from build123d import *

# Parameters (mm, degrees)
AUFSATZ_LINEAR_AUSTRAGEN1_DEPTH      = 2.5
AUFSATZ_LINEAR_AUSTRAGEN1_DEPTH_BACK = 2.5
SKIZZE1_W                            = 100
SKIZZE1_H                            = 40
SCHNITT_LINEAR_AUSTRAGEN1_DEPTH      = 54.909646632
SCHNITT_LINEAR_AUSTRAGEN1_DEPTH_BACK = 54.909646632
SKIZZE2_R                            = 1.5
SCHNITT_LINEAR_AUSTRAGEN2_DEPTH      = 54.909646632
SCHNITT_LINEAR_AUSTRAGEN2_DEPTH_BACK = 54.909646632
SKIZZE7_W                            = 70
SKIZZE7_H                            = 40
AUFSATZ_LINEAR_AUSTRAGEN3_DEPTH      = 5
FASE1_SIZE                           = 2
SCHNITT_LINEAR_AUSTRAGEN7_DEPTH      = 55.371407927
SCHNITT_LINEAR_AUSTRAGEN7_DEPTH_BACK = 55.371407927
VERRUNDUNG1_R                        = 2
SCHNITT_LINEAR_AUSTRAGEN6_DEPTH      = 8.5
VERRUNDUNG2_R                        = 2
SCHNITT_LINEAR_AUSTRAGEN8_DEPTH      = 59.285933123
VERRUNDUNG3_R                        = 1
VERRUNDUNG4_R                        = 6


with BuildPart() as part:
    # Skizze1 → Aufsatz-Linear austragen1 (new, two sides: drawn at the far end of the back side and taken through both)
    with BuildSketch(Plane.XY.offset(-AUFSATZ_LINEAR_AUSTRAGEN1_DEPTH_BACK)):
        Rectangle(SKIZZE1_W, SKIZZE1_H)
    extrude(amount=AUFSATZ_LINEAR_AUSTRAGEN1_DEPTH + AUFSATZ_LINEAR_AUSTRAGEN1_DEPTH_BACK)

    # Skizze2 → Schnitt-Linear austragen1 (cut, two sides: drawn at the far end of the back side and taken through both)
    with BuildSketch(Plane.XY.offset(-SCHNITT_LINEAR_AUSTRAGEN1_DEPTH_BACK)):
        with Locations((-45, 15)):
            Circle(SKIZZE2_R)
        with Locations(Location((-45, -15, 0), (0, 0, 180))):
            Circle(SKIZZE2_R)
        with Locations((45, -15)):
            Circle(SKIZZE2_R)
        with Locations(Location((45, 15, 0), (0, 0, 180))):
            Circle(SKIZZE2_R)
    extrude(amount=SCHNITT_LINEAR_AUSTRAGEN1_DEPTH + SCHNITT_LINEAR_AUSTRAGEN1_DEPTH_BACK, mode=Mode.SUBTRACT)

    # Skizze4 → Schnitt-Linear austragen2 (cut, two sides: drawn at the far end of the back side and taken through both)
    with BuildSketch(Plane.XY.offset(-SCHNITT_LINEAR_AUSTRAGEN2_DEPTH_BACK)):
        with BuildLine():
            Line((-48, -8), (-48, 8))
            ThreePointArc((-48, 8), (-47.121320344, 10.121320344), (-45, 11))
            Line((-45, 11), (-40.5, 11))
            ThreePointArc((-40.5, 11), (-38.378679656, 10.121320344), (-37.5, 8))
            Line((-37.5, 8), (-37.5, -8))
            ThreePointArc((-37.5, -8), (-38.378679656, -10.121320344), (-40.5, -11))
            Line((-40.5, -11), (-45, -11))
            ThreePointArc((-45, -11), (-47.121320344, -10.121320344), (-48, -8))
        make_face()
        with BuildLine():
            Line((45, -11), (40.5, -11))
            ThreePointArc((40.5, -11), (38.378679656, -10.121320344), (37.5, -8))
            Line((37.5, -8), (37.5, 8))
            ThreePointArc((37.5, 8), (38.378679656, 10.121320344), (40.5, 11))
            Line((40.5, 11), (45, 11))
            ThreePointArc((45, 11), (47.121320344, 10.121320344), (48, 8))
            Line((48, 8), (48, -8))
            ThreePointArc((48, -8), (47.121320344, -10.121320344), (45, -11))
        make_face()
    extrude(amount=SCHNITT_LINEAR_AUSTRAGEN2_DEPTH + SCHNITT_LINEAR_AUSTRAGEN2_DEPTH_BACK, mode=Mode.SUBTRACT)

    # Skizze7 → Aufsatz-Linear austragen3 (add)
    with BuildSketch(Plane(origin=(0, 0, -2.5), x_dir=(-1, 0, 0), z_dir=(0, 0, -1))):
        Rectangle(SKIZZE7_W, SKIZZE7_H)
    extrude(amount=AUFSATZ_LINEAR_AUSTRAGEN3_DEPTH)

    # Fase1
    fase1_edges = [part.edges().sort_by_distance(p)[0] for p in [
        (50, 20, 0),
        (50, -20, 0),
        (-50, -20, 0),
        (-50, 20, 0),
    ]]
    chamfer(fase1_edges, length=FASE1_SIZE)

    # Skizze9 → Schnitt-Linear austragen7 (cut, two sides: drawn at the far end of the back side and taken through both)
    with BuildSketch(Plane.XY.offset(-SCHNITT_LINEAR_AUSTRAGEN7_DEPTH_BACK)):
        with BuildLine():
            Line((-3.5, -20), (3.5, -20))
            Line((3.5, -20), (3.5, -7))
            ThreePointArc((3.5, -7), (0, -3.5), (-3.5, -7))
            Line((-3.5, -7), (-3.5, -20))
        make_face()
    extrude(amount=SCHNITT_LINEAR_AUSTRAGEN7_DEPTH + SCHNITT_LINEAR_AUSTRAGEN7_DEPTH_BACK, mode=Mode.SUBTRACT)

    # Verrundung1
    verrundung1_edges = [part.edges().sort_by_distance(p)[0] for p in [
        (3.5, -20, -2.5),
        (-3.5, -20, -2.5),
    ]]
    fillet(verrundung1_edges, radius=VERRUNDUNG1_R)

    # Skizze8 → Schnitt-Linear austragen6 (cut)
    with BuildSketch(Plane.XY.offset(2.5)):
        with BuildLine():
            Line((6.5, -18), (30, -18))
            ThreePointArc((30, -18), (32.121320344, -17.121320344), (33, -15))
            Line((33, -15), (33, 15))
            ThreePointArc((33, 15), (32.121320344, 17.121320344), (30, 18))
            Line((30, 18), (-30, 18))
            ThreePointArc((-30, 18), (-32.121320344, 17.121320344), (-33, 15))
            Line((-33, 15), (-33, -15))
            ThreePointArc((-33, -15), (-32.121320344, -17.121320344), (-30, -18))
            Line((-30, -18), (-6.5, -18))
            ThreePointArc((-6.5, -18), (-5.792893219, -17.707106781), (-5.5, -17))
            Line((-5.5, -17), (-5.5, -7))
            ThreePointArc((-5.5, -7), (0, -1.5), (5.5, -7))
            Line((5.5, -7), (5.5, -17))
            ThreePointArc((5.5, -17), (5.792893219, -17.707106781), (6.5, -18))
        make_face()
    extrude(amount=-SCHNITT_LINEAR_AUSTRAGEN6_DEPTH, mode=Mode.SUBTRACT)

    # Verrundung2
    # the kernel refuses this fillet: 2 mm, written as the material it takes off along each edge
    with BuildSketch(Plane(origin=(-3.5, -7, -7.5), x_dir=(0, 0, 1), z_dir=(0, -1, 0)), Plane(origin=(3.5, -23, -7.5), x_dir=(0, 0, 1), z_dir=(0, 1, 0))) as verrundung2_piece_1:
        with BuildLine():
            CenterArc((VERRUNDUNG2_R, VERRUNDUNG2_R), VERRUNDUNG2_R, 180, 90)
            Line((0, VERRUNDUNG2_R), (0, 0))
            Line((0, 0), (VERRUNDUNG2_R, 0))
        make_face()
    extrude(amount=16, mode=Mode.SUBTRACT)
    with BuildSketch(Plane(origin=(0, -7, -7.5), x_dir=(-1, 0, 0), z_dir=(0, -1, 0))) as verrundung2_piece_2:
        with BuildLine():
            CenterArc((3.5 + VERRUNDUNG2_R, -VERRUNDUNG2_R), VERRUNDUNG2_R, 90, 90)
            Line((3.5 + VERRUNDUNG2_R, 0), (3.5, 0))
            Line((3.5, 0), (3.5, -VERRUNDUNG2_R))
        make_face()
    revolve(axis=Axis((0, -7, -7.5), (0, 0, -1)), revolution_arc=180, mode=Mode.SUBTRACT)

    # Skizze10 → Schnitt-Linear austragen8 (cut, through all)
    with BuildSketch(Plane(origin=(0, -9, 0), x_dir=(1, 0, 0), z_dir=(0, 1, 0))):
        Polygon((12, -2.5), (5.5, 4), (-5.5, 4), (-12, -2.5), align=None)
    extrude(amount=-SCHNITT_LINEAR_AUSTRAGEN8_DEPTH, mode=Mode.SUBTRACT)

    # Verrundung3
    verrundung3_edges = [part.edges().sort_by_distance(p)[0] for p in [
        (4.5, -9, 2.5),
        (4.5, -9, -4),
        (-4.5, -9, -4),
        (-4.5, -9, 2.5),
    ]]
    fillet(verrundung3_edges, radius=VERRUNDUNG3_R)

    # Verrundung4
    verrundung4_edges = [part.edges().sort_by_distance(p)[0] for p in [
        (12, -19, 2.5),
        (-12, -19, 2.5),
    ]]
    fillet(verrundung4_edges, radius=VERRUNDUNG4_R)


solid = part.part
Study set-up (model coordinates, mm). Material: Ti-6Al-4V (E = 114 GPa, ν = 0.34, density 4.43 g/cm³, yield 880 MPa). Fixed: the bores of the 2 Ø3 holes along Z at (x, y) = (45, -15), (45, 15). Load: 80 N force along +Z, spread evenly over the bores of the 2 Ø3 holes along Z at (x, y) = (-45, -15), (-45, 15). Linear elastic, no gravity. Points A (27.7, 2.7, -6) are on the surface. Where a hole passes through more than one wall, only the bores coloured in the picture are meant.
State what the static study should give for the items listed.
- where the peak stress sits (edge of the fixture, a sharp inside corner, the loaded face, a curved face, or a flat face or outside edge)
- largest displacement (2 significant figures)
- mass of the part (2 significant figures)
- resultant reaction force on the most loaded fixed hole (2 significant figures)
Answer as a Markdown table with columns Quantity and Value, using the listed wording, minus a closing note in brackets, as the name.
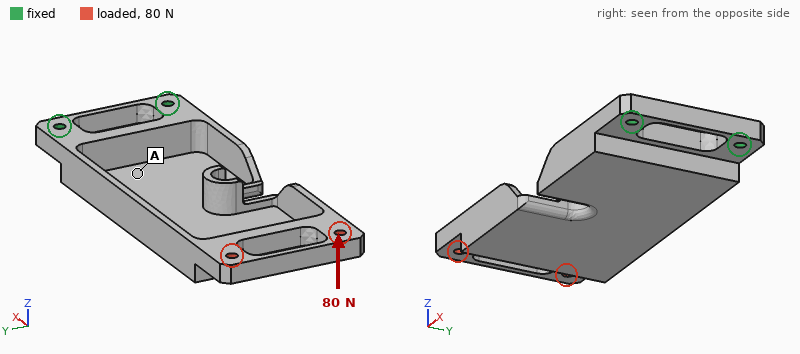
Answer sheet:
| Quantity | Value |
|---|---|
| where the peak stress sits | a curved face |
| largest displacement | 1.1 mm |
| mass of the part | 50 g |
| resultant reaction force on the most loaded fixed hole | 150 N |
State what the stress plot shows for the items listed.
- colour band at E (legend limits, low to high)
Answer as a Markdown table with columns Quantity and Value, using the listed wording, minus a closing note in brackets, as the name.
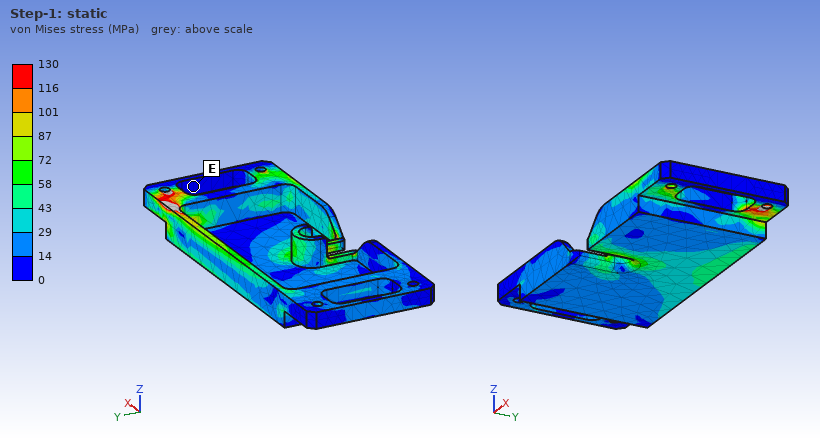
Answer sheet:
| Quantity | Value |
|---|---|
| colour band at E | 0 to 14 MPa |
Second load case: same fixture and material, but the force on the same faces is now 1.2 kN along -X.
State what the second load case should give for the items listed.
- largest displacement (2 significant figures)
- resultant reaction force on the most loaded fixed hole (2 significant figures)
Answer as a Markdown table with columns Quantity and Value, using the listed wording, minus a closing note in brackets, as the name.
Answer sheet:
| Quantity | Value |
|---|---|
| largest displacement | 1.3 mm |
| resultant reaction force on the most loaded fixed hole | 620 N |
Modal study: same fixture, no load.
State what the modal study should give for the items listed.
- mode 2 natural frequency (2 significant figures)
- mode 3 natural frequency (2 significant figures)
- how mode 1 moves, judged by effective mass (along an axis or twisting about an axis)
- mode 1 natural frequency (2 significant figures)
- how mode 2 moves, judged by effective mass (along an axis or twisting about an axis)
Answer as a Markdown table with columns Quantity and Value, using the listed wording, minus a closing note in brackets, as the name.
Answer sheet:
| Quantity | Value |
|---|---|
| mode 2 natural frequency | 790 Hz |
| mode 3 natural frequency | 1800 Hz |
| how mode 1 moves, judged by effective mass | along Z |
| mode 1 natural frequency | 390 Hz |
| how mode 2 moves, judged by effective mass | along Y |
